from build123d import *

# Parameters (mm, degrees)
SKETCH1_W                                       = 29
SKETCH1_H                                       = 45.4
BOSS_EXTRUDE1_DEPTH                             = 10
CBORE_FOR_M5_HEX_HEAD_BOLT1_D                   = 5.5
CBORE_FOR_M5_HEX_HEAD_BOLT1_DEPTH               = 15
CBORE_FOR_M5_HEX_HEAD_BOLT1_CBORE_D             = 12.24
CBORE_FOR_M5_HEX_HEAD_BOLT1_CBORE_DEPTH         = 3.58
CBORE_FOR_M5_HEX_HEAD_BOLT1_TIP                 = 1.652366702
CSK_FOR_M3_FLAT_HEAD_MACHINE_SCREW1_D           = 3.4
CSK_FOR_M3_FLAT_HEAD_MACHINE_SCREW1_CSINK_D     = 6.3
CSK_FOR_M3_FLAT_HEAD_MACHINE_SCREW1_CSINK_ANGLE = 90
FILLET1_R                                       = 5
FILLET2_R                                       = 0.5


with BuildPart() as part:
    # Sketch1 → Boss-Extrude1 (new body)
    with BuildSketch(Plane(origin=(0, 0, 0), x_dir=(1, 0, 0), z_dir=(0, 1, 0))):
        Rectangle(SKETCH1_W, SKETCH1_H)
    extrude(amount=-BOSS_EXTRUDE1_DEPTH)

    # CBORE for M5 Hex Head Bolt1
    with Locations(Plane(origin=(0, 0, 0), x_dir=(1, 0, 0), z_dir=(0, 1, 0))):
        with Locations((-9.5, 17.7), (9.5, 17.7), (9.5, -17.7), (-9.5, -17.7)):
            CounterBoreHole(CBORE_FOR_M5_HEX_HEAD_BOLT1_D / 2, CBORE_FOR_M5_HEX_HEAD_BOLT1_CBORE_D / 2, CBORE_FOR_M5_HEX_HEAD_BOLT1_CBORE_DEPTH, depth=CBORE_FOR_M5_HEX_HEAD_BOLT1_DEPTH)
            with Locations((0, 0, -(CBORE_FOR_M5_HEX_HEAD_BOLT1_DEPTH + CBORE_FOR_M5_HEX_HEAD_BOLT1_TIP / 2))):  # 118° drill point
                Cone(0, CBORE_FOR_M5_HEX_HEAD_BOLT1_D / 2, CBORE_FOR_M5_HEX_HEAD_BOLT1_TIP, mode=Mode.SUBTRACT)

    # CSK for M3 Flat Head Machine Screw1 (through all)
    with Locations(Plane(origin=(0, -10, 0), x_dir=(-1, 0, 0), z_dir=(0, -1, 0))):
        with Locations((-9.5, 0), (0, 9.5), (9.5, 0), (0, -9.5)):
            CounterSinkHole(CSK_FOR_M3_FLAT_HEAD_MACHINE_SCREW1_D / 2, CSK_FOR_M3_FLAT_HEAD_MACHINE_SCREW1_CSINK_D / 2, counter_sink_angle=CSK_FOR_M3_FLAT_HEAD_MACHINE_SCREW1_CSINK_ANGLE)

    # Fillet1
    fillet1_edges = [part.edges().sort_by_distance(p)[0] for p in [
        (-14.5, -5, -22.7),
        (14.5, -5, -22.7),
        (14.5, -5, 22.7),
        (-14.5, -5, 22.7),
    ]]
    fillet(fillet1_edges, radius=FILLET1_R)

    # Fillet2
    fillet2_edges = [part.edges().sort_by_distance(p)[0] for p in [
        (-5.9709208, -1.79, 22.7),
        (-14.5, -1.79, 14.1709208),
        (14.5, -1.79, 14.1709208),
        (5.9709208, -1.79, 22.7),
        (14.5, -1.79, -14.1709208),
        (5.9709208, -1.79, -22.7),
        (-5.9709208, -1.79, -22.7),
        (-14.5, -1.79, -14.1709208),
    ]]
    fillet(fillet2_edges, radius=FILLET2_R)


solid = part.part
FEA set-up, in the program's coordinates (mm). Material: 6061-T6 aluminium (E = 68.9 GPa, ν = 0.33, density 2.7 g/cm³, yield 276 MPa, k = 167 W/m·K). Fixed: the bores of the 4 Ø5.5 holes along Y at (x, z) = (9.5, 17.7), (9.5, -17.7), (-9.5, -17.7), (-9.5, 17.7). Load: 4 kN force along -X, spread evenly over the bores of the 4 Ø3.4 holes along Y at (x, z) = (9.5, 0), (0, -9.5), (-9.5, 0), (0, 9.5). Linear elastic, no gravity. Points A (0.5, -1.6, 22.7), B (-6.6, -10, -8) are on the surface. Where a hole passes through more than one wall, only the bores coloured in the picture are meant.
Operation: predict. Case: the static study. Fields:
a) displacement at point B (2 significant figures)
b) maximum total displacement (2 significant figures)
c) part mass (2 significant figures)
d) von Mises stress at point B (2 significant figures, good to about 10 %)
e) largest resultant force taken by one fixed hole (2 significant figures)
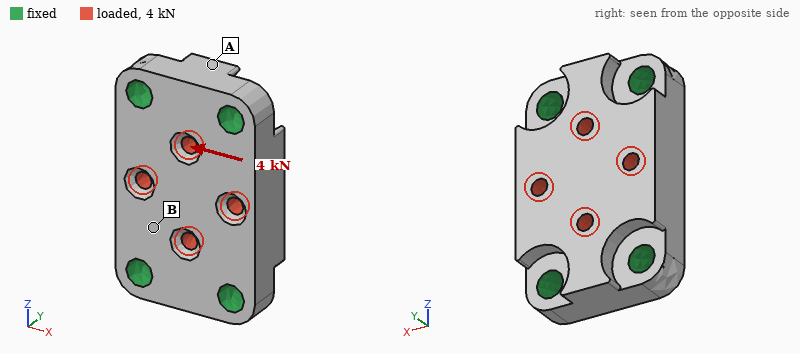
3.2 µm
6.7 µm
28 g
11 MPa
1.2 kN
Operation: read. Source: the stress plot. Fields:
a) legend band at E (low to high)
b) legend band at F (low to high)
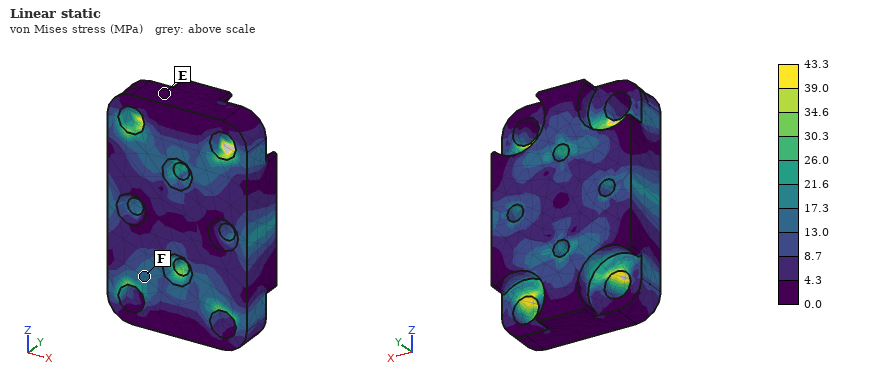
0.0 to 4.3 MPa
13.0 to 17.3 MPa
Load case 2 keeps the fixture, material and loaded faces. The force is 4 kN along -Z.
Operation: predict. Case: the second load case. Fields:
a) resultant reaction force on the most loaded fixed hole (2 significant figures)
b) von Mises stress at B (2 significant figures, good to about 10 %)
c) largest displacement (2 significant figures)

1.0 kN
8.0 MPa
2.5 µm
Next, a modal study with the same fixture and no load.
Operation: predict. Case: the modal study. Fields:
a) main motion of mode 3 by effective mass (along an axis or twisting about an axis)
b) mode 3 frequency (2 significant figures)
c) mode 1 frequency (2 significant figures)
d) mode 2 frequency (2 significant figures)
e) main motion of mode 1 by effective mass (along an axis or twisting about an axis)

along X
37 kHz
26 kHz
32 kHz
along Y
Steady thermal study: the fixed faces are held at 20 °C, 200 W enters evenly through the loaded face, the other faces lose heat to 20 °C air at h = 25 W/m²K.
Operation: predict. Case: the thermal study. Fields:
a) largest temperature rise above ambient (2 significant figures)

35 K
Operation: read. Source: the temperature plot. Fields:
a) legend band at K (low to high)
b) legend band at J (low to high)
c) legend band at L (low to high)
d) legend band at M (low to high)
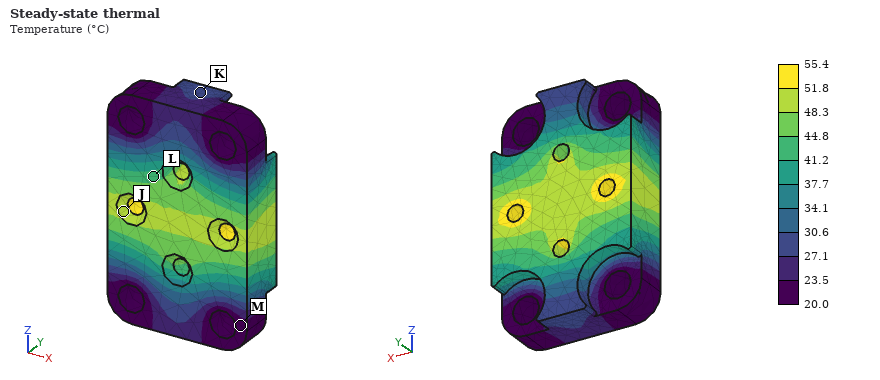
27.1 to 30.6 °C
48.3 to 51.8 °C
41.2 to 44.8 °C
20.0 to 23.5 °C
